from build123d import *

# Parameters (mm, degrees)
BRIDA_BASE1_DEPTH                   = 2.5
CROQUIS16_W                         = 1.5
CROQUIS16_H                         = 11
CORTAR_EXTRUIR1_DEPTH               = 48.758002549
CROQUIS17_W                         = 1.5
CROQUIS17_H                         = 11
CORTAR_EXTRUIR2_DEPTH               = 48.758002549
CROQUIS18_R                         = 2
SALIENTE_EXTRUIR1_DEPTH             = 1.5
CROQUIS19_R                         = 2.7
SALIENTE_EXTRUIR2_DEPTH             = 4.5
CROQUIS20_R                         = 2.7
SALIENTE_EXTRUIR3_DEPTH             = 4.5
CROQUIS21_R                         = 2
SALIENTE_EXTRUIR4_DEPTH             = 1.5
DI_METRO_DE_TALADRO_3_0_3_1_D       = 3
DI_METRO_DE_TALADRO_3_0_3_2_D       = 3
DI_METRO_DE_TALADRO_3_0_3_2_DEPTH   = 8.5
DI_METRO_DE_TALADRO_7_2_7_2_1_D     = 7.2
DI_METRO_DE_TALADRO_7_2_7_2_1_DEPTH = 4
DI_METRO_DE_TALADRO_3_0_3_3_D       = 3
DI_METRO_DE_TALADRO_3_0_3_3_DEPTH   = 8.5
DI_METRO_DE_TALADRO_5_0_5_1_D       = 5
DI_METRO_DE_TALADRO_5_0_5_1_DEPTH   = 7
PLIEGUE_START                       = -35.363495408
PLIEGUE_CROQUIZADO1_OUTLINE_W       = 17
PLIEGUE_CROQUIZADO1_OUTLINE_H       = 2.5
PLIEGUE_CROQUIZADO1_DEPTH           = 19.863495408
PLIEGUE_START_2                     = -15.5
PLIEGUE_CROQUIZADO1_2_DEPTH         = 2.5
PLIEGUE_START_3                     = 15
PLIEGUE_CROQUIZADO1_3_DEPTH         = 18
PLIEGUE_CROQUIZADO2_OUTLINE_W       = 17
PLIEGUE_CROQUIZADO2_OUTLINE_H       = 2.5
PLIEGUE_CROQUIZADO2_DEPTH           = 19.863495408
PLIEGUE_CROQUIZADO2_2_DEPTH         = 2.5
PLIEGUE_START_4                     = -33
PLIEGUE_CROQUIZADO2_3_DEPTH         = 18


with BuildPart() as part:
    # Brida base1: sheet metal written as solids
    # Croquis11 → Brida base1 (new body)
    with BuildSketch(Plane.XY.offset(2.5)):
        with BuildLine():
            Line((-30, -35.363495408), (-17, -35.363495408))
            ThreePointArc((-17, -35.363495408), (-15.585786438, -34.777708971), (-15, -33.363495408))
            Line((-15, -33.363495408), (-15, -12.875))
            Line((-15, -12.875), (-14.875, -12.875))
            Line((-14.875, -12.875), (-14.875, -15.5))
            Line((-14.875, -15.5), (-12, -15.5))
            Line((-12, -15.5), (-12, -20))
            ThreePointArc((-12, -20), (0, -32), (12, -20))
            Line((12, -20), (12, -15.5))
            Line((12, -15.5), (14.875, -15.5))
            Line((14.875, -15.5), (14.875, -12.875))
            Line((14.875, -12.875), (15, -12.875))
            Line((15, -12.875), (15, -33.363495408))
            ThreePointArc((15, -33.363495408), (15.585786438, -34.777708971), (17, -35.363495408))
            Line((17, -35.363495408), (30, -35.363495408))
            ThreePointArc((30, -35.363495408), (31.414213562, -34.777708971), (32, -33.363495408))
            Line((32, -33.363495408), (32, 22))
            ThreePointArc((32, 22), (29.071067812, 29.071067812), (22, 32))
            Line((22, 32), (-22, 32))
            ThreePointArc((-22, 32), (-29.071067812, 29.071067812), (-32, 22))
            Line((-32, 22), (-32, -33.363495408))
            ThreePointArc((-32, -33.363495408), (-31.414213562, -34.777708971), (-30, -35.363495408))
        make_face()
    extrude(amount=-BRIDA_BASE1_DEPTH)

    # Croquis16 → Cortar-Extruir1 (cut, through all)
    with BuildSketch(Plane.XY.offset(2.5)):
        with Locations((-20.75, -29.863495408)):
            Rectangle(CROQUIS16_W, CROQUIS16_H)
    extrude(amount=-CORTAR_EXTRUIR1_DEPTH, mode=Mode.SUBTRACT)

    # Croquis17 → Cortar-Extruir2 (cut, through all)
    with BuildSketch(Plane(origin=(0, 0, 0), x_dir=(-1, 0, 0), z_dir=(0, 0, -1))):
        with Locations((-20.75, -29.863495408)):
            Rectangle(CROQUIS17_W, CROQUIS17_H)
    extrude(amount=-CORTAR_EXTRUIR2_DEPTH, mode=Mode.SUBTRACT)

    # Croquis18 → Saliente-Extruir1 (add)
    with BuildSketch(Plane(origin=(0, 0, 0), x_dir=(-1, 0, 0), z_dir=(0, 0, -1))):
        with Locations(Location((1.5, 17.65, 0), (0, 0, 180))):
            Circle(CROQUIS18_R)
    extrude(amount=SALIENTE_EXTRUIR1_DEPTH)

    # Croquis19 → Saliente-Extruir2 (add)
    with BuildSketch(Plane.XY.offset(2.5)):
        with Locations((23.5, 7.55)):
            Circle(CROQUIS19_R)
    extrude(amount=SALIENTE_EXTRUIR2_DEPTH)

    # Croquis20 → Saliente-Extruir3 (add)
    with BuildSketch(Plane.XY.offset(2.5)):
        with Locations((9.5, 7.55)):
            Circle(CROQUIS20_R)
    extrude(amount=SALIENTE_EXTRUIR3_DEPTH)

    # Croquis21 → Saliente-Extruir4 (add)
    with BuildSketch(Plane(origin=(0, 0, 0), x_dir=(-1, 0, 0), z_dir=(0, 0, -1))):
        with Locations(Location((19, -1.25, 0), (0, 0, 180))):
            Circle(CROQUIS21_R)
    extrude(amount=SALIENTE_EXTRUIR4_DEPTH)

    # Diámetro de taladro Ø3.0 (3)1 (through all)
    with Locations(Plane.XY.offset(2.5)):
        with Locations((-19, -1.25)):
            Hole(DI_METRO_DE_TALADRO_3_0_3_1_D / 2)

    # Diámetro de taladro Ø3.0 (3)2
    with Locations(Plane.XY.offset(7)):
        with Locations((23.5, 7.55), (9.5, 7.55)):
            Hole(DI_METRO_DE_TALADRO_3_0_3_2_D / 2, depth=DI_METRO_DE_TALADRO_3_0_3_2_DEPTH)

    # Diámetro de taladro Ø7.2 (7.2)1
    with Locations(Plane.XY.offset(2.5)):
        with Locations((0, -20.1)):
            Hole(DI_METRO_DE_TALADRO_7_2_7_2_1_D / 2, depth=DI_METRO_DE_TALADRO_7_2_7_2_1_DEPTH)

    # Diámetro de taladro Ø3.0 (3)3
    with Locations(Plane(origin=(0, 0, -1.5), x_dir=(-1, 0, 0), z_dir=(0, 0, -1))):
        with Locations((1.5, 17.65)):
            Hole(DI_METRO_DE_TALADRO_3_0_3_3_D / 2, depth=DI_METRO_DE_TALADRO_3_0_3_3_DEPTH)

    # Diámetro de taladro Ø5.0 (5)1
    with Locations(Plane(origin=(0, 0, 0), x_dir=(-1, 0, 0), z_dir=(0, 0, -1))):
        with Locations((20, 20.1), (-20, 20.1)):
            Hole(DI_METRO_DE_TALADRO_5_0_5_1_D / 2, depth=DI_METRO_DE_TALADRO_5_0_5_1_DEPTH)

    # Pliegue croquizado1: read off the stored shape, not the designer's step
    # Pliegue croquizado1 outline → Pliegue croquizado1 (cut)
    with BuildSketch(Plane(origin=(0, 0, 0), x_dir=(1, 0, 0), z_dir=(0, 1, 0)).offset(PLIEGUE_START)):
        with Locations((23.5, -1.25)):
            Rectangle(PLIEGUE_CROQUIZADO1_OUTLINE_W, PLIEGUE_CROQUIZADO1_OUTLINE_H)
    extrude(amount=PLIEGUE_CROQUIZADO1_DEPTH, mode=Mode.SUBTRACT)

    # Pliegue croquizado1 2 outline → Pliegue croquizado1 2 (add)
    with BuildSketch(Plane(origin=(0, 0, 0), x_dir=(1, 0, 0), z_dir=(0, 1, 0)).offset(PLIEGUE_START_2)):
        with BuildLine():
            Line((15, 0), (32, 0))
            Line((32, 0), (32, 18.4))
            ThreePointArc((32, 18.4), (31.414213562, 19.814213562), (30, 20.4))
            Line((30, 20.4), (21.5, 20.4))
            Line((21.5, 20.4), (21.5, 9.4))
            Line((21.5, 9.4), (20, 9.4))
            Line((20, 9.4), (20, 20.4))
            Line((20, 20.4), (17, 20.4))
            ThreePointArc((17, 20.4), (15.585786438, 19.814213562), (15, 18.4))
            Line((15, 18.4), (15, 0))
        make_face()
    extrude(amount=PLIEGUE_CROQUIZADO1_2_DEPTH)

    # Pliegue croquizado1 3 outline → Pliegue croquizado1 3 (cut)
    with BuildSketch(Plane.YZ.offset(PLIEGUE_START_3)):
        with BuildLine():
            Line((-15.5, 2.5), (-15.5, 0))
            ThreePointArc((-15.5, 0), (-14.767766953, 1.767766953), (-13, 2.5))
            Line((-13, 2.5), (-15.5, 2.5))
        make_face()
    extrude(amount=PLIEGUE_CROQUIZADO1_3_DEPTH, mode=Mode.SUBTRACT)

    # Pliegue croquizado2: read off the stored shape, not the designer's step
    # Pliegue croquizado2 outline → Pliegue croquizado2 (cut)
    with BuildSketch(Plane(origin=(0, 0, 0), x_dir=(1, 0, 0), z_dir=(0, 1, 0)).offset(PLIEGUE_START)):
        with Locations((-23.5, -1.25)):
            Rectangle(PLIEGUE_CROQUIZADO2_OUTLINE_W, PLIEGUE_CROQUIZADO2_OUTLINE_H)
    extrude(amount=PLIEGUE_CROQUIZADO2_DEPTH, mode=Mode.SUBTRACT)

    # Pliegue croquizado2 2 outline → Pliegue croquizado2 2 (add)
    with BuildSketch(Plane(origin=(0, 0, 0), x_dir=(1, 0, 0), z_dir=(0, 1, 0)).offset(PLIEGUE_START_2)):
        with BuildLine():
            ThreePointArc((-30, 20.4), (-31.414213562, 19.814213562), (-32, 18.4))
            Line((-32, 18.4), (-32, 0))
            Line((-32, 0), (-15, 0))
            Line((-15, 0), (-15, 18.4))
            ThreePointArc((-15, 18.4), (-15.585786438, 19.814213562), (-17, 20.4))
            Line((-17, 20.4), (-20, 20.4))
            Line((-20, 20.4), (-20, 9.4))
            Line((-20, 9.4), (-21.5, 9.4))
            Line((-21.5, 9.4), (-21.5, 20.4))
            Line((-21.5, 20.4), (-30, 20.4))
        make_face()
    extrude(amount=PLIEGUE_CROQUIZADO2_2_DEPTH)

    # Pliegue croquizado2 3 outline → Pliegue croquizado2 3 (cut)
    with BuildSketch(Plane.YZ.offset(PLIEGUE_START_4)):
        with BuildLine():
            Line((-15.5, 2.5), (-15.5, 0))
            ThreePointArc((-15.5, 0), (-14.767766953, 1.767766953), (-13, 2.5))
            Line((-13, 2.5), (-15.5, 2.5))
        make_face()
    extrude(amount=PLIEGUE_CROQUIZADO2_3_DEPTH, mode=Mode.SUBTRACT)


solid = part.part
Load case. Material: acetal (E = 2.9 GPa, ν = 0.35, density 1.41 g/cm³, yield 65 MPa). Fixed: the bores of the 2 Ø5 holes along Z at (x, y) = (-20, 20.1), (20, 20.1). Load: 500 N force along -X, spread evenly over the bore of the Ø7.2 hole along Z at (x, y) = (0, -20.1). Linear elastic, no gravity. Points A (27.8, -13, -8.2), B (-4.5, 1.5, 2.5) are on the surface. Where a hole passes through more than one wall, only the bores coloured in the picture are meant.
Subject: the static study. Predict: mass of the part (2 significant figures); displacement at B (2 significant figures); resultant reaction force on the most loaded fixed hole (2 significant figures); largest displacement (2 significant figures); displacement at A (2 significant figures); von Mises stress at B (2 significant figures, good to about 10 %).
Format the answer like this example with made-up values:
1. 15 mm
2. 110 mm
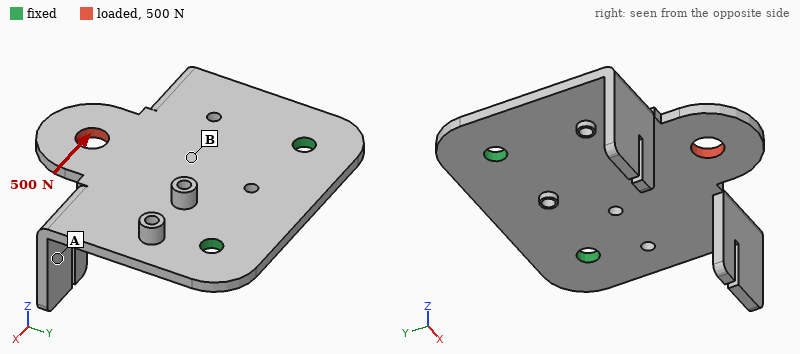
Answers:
1. 14 g
2. 0.10 mm
3. 530 N
4. 0.42 mm
5. 0.21 mm
6. 7.0 MPa
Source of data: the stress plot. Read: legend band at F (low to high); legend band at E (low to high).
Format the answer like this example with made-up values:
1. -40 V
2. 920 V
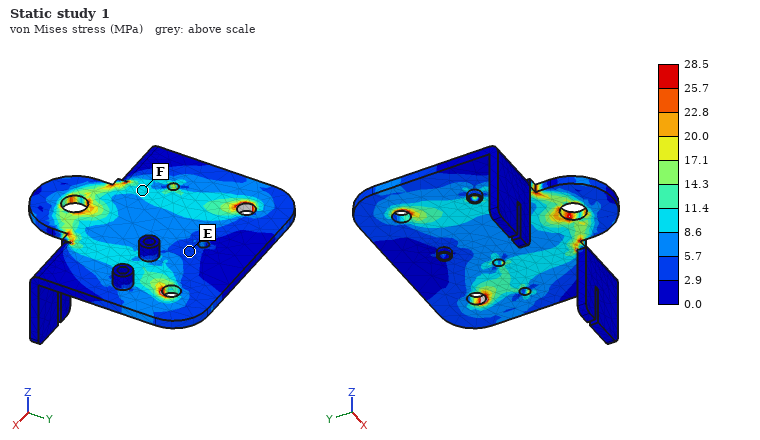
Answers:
1. 8.6 to 11.4 MPa
2. 2.9 to 5.7 MPa
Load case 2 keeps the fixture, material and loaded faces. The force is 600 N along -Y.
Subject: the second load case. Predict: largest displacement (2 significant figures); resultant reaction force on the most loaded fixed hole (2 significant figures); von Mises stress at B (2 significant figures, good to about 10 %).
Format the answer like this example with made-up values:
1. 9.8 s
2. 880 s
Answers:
1. 0.15 mm
2. 310 N
3. 6.0 MPa
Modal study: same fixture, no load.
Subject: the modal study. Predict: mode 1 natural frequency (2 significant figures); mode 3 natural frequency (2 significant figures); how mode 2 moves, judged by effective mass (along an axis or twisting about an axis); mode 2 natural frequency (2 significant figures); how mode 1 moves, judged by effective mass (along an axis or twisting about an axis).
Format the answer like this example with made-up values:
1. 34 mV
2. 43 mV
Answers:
1. 250 Hz
2. 640 Hz
3. twisting about Y
4. 410 Hz
5. along Z
